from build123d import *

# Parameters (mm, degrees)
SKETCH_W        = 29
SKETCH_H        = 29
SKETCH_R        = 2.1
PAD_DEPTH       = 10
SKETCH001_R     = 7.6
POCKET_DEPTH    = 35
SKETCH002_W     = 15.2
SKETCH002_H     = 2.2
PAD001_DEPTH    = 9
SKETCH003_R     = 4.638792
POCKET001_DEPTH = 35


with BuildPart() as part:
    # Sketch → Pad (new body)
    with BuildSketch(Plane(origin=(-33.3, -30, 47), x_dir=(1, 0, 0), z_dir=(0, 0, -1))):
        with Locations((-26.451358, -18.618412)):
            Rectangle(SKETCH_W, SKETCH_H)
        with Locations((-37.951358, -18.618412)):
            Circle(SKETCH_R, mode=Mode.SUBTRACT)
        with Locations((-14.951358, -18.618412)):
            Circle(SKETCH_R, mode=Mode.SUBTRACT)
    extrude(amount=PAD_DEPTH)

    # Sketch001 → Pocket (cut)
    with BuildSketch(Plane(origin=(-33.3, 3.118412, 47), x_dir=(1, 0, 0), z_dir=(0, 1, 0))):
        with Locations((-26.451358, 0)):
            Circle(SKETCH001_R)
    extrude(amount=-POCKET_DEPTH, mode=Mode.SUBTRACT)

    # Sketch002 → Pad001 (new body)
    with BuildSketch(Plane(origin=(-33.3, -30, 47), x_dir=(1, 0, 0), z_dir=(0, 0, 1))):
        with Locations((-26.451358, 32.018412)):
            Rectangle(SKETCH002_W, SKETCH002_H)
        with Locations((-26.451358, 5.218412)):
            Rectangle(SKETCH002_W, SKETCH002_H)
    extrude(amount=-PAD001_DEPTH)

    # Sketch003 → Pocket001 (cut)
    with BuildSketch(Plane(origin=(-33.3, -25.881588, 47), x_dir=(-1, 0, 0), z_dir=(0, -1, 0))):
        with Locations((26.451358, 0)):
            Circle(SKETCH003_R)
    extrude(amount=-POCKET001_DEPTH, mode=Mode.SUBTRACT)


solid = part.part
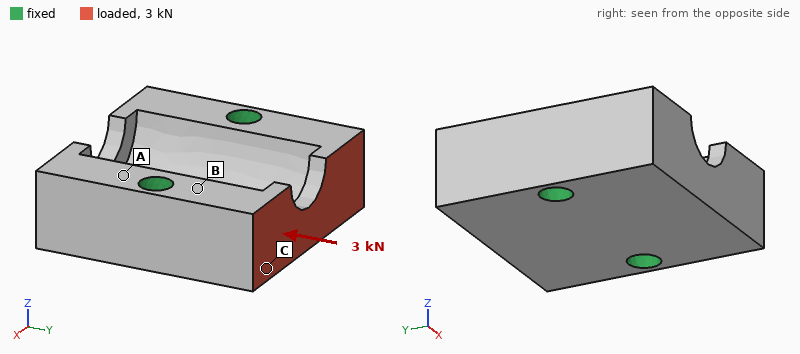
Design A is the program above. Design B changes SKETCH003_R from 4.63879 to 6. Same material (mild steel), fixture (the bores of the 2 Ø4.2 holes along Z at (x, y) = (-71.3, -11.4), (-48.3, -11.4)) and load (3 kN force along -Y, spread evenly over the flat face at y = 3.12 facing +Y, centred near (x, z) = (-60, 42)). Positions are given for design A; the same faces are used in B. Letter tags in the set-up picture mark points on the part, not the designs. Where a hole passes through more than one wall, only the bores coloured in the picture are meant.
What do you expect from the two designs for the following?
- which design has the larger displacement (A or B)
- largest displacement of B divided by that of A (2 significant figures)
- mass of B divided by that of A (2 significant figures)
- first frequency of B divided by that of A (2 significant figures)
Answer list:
A
0.55
0.98
1.0
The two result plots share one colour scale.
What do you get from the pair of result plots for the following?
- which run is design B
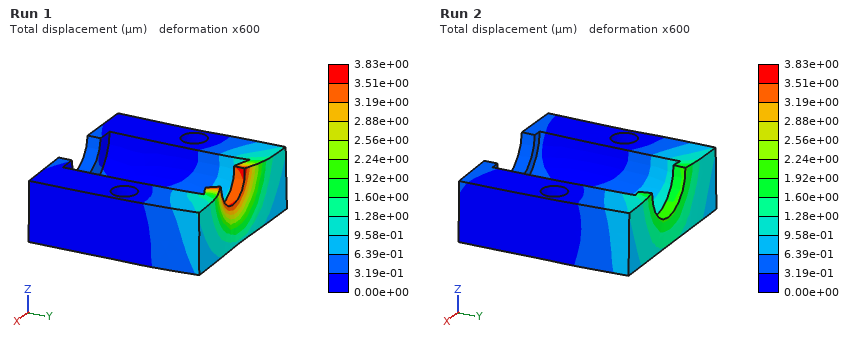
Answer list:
Run 2
